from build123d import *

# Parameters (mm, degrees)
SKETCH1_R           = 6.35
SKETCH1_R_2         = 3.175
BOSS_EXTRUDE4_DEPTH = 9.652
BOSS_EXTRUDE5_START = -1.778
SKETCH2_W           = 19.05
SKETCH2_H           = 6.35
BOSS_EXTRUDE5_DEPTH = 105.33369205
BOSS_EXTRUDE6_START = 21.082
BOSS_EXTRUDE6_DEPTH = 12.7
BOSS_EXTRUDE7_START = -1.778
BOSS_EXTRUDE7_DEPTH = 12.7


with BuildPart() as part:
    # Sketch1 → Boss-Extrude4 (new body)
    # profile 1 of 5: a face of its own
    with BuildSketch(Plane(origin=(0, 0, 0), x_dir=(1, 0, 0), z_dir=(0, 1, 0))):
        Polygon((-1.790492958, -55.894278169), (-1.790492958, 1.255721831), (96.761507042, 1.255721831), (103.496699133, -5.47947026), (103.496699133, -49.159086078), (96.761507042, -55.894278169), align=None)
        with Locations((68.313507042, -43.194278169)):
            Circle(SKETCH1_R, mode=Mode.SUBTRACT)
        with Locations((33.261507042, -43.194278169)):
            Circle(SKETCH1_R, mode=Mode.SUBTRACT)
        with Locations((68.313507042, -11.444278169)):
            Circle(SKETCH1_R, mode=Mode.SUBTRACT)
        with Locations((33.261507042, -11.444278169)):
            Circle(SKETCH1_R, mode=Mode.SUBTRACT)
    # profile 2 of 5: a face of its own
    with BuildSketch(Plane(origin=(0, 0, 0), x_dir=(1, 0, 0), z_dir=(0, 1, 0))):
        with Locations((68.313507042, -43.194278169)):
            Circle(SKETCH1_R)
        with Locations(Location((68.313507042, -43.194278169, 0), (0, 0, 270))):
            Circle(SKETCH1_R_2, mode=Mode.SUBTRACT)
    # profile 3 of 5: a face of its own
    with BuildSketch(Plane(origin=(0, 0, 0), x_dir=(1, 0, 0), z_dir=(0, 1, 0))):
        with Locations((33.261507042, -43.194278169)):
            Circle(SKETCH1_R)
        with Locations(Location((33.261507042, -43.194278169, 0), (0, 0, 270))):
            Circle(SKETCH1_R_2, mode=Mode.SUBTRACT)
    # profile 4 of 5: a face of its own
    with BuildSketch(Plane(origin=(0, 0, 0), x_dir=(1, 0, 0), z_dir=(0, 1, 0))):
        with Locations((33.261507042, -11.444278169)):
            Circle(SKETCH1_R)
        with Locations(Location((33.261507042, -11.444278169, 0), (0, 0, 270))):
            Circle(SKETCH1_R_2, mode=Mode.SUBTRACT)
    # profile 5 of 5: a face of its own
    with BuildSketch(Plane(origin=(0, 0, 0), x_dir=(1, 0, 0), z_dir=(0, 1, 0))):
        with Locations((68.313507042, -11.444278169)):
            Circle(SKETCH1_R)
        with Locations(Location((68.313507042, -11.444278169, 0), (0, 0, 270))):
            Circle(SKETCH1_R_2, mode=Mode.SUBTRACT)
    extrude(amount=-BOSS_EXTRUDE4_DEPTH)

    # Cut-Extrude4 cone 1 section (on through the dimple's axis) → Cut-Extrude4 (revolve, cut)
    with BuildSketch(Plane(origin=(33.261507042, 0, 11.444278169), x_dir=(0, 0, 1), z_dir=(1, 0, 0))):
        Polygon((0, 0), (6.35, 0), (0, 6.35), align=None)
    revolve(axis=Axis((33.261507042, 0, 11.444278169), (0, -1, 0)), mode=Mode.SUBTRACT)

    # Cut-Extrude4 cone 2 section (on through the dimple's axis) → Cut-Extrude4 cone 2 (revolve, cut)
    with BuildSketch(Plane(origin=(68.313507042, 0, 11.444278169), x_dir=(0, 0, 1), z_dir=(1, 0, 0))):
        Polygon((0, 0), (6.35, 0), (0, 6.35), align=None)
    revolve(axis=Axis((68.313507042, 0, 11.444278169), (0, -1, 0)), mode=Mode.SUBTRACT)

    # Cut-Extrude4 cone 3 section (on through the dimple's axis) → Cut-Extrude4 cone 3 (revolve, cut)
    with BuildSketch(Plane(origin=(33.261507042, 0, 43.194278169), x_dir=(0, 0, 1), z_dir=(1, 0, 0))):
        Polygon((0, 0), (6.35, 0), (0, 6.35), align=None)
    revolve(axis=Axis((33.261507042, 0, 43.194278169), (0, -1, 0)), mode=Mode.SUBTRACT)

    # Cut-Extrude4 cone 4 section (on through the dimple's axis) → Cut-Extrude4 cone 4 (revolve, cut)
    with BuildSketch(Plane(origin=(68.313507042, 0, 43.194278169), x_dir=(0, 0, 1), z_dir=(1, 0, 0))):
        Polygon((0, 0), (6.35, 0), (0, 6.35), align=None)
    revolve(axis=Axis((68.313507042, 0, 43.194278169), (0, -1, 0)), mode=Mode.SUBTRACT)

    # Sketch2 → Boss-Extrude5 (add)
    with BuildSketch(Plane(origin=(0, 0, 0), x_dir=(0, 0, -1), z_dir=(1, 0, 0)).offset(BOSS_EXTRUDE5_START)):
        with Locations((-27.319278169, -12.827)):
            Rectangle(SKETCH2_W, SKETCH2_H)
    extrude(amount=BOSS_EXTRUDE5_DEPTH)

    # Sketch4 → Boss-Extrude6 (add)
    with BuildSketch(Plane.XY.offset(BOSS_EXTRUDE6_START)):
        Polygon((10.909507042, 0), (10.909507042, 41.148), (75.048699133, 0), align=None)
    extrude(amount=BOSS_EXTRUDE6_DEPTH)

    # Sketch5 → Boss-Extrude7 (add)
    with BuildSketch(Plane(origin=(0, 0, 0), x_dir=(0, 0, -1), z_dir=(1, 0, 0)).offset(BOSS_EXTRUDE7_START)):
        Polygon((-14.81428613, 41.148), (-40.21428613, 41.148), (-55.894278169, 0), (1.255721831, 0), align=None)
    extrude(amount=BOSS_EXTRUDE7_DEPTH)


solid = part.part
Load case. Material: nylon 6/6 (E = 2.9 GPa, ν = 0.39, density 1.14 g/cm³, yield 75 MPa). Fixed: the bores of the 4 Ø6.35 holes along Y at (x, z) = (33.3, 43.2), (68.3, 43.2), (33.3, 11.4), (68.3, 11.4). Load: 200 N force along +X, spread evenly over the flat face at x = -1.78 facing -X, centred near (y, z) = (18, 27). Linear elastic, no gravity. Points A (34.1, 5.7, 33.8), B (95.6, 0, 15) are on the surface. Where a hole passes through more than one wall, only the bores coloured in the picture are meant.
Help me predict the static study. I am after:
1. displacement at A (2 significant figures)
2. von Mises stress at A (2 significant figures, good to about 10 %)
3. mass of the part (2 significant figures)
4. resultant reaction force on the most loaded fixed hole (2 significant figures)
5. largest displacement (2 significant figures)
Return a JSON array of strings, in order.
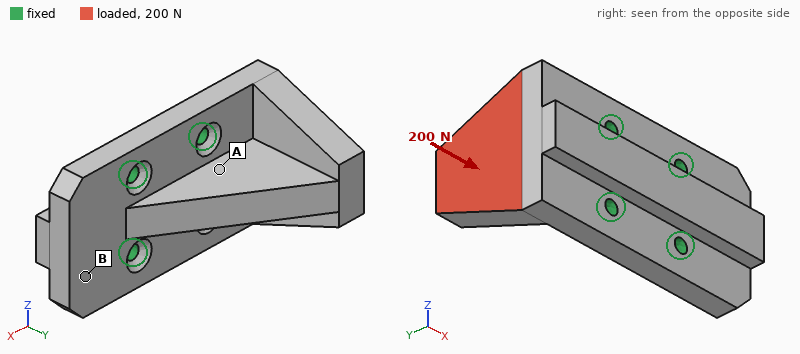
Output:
["9.5 µm", "0.59 MPa", "120 g", "77 N", "54 µm"]
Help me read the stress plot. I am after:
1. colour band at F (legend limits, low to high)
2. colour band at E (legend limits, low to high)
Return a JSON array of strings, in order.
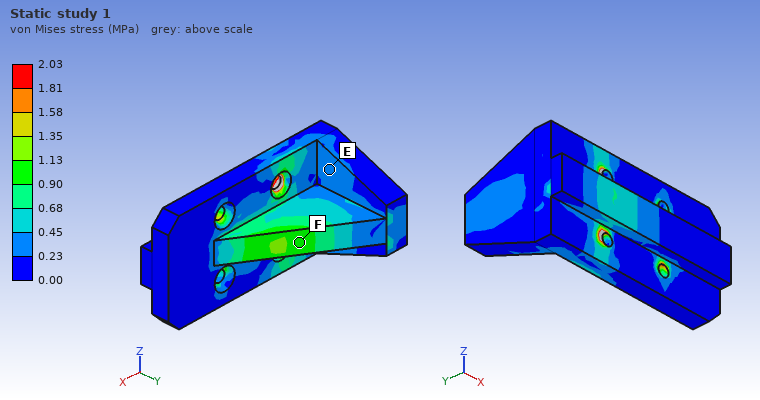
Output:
["0.90 to 1.13 MPa", "0.23 to 0.45 MPa"]
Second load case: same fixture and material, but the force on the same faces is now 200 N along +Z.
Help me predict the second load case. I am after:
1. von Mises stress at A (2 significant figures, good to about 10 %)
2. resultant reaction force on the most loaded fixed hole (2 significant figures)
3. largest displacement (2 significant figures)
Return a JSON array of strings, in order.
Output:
["1.1 MPa", "230 N", "96 µm"]
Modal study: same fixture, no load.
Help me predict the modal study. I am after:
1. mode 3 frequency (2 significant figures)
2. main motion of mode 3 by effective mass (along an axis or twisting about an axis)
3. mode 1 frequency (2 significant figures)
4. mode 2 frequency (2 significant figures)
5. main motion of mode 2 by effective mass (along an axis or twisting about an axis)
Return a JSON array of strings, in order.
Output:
["2100 Hz", "along Y", "1400 Hz", "1500 Hz", "along Z"]
